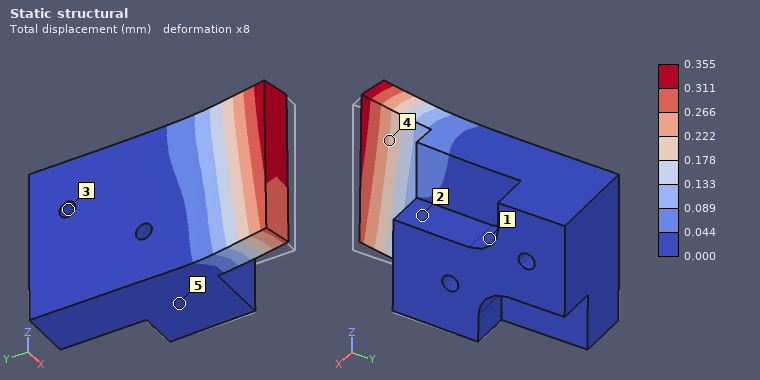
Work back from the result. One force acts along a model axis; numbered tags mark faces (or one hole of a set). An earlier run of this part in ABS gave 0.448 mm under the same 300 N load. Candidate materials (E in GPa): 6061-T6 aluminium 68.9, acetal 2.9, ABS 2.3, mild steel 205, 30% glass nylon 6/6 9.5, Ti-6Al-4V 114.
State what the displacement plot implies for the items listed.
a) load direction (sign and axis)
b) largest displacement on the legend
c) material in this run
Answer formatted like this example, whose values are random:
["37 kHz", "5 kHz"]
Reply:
["-X", "0.355 mm", "acetal"]
